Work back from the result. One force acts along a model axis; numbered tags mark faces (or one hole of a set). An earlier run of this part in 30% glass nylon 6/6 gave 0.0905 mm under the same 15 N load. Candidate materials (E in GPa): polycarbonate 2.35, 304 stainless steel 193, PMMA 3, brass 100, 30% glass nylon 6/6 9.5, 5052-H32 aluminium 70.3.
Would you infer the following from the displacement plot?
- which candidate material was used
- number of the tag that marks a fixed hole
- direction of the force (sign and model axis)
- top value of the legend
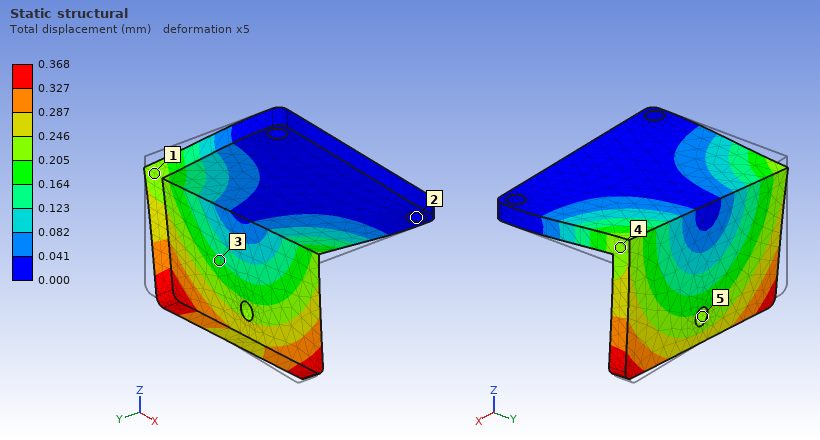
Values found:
polycarbonate
2
+X
0.368 mm
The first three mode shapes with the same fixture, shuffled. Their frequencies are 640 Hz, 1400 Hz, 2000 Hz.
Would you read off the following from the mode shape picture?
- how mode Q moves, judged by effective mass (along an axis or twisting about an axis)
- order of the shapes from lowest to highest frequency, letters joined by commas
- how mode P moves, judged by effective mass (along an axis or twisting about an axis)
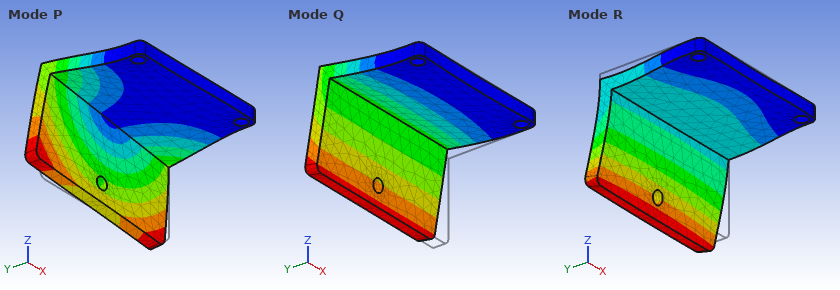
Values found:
along Z
Q, P, R
along X
